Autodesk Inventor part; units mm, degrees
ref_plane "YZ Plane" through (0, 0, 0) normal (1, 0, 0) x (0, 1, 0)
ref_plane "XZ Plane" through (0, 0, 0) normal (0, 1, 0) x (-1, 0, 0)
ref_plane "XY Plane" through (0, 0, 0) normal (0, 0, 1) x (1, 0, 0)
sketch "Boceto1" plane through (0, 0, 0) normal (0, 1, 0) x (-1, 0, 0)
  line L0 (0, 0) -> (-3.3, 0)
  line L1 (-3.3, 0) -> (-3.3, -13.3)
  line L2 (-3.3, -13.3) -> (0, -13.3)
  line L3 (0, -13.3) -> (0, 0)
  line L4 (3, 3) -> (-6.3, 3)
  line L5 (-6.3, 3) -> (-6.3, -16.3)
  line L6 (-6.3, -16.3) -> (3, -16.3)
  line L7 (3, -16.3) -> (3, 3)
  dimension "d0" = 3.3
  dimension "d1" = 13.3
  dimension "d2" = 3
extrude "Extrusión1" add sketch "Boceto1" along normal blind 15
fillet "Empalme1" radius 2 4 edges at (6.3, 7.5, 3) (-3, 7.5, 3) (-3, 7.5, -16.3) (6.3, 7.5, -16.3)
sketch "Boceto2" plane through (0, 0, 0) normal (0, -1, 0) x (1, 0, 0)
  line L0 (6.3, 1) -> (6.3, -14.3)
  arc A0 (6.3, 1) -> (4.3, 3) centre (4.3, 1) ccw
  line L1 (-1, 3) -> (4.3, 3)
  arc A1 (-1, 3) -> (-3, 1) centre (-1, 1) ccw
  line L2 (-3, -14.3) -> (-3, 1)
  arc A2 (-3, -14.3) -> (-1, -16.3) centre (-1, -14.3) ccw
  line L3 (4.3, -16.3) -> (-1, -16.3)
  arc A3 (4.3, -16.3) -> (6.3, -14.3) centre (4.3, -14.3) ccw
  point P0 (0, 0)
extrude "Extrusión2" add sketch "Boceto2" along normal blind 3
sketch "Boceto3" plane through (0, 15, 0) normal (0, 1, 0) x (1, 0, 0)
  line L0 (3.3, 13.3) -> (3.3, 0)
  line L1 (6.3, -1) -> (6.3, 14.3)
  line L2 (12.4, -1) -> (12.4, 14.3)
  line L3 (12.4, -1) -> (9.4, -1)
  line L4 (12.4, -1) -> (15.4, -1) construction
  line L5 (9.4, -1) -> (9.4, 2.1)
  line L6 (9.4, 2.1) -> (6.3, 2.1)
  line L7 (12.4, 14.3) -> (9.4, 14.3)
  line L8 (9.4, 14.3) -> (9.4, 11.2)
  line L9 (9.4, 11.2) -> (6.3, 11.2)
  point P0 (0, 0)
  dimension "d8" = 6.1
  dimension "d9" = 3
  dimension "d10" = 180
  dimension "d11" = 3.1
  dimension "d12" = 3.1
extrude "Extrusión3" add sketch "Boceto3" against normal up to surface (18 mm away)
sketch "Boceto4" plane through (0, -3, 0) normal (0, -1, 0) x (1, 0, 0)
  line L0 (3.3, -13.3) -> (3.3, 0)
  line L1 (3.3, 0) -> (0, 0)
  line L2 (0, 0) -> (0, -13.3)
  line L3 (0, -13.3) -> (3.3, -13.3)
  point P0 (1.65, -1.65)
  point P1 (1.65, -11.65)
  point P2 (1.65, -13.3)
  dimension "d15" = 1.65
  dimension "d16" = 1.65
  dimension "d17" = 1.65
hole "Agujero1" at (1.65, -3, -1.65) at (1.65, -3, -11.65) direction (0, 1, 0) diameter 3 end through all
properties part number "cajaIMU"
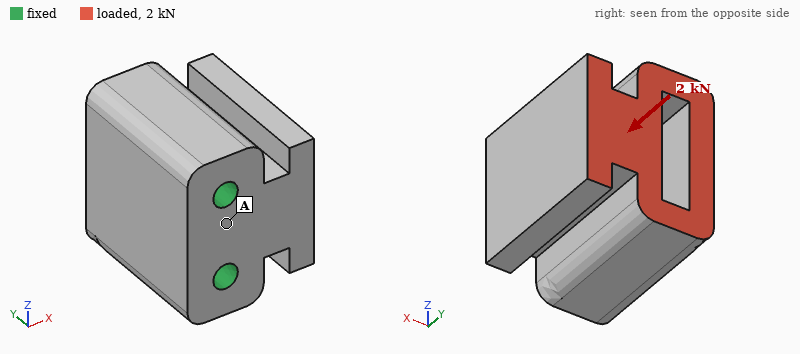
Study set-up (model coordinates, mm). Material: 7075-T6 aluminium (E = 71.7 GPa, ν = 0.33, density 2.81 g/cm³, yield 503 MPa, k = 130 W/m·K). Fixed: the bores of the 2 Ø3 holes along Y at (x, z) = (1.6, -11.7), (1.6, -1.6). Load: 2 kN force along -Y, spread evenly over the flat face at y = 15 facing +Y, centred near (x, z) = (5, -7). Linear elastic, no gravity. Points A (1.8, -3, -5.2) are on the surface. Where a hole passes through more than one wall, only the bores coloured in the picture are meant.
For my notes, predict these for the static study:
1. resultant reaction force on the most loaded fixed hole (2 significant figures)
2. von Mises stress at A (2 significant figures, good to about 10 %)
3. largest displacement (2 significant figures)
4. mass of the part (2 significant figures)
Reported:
1.0 kN
31 MPa
39 µm
11 g
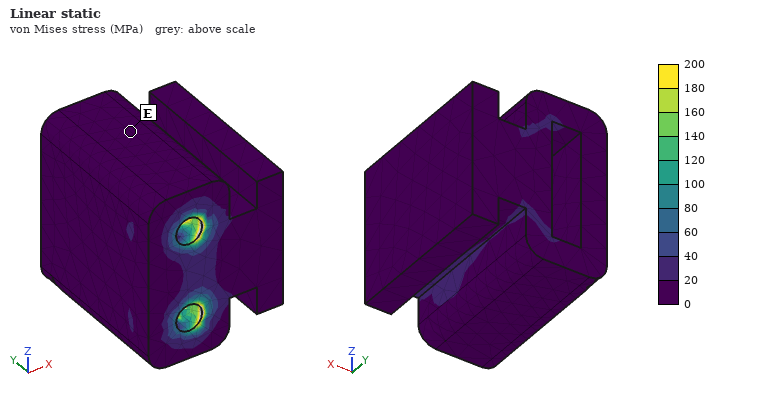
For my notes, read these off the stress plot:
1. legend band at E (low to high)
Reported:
0 to 20 MPa
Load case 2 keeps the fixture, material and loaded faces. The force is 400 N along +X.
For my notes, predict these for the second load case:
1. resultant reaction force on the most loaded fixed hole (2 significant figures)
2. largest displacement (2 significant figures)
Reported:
200 N
43 µm
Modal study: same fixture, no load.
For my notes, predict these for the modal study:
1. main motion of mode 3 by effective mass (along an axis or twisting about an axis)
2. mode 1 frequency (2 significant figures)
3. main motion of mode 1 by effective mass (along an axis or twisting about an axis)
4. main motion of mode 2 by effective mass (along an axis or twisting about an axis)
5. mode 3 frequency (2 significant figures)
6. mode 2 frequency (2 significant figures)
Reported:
twisting about Y
8400 Hz
along X
along Z
26 kHz
19 kHz
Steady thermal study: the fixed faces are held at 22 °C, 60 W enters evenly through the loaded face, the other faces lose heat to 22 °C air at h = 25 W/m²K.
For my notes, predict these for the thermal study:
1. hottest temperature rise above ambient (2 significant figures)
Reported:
51 K
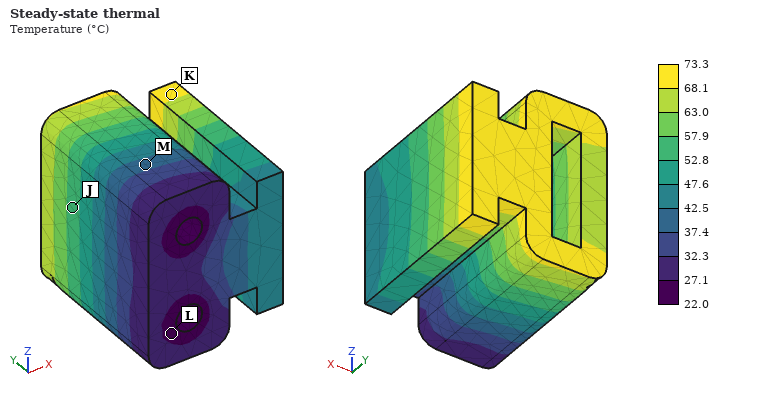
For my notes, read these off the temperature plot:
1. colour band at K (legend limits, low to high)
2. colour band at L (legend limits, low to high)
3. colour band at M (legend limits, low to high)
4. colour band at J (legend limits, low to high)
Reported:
68.1 to 73.3 °C
22.0 to 27.1 °C
37.4 to 42.5 °C
52.8 to 57.9 °C
